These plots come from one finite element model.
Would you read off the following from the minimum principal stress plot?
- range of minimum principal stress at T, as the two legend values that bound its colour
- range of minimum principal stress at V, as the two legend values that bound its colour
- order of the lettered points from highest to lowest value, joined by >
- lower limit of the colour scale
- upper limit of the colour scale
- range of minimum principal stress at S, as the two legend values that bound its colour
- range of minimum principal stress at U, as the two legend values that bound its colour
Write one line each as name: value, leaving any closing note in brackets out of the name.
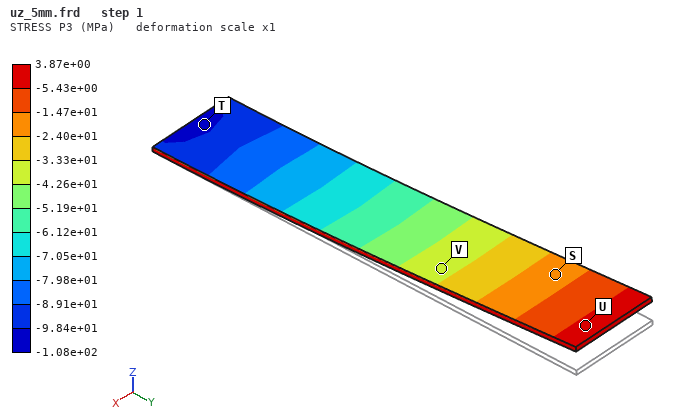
range of minimum principal stress at T, as the two legend values that bound its colour: -1.08e+02 to -9.84e+01 MPa
range of minimum principal stress at V, as the two legend values that bound its colour: -4.26e+01 to -3.33e+01 MPa
order of the lettered points from highest to lowest value, joined by >: U > S > V > T
lower limit of the colour scale: -1.08e+02 MPa
upper limit of the colour scale: 3.87e+00 MPa
range of minimum principal stress at S, as the two legend values that bound its colour: -2.40e+01 to -1.47e+01 MPa
range of minimum principal stress at U, as the two legend values that bound its colour: -5.43e+00 to 3.87e+00 MPa
